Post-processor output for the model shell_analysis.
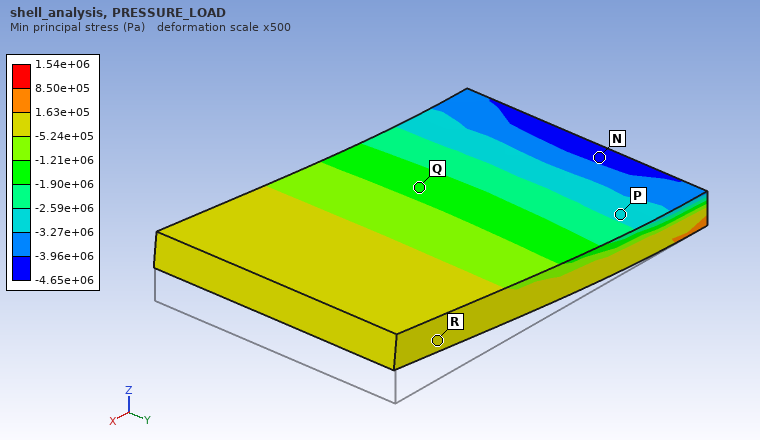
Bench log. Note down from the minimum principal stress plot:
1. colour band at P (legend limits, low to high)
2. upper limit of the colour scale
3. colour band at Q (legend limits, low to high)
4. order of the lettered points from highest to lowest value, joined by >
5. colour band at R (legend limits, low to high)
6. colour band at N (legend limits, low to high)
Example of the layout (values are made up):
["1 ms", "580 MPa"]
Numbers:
["-3.27e+06 to -2.59e+06 Pa", "1.54e+06 Pa", "-1.90e+06 to -1.21e+06 Pa", "R > Q > P > N", "-5.24e+05 to 1.63e+05 Pa", "-4.65e+06 to -3.96e+06 Pa"]
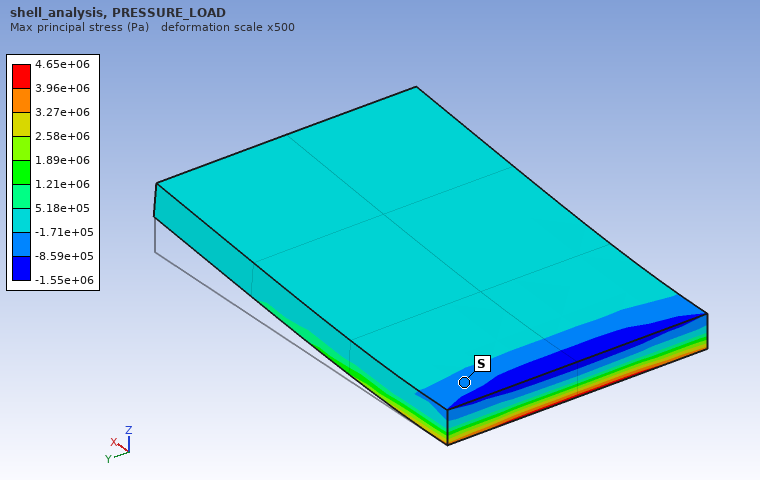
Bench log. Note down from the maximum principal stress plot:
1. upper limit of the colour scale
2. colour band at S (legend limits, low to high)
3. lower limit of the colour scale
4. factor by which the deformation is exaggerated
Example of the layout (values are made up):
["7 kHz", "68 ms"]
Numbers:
["4.65e+06 Pa", "-8.59e+05 to -1.71e+05 Pa", "-1.55e+06 Pa", "500"]
